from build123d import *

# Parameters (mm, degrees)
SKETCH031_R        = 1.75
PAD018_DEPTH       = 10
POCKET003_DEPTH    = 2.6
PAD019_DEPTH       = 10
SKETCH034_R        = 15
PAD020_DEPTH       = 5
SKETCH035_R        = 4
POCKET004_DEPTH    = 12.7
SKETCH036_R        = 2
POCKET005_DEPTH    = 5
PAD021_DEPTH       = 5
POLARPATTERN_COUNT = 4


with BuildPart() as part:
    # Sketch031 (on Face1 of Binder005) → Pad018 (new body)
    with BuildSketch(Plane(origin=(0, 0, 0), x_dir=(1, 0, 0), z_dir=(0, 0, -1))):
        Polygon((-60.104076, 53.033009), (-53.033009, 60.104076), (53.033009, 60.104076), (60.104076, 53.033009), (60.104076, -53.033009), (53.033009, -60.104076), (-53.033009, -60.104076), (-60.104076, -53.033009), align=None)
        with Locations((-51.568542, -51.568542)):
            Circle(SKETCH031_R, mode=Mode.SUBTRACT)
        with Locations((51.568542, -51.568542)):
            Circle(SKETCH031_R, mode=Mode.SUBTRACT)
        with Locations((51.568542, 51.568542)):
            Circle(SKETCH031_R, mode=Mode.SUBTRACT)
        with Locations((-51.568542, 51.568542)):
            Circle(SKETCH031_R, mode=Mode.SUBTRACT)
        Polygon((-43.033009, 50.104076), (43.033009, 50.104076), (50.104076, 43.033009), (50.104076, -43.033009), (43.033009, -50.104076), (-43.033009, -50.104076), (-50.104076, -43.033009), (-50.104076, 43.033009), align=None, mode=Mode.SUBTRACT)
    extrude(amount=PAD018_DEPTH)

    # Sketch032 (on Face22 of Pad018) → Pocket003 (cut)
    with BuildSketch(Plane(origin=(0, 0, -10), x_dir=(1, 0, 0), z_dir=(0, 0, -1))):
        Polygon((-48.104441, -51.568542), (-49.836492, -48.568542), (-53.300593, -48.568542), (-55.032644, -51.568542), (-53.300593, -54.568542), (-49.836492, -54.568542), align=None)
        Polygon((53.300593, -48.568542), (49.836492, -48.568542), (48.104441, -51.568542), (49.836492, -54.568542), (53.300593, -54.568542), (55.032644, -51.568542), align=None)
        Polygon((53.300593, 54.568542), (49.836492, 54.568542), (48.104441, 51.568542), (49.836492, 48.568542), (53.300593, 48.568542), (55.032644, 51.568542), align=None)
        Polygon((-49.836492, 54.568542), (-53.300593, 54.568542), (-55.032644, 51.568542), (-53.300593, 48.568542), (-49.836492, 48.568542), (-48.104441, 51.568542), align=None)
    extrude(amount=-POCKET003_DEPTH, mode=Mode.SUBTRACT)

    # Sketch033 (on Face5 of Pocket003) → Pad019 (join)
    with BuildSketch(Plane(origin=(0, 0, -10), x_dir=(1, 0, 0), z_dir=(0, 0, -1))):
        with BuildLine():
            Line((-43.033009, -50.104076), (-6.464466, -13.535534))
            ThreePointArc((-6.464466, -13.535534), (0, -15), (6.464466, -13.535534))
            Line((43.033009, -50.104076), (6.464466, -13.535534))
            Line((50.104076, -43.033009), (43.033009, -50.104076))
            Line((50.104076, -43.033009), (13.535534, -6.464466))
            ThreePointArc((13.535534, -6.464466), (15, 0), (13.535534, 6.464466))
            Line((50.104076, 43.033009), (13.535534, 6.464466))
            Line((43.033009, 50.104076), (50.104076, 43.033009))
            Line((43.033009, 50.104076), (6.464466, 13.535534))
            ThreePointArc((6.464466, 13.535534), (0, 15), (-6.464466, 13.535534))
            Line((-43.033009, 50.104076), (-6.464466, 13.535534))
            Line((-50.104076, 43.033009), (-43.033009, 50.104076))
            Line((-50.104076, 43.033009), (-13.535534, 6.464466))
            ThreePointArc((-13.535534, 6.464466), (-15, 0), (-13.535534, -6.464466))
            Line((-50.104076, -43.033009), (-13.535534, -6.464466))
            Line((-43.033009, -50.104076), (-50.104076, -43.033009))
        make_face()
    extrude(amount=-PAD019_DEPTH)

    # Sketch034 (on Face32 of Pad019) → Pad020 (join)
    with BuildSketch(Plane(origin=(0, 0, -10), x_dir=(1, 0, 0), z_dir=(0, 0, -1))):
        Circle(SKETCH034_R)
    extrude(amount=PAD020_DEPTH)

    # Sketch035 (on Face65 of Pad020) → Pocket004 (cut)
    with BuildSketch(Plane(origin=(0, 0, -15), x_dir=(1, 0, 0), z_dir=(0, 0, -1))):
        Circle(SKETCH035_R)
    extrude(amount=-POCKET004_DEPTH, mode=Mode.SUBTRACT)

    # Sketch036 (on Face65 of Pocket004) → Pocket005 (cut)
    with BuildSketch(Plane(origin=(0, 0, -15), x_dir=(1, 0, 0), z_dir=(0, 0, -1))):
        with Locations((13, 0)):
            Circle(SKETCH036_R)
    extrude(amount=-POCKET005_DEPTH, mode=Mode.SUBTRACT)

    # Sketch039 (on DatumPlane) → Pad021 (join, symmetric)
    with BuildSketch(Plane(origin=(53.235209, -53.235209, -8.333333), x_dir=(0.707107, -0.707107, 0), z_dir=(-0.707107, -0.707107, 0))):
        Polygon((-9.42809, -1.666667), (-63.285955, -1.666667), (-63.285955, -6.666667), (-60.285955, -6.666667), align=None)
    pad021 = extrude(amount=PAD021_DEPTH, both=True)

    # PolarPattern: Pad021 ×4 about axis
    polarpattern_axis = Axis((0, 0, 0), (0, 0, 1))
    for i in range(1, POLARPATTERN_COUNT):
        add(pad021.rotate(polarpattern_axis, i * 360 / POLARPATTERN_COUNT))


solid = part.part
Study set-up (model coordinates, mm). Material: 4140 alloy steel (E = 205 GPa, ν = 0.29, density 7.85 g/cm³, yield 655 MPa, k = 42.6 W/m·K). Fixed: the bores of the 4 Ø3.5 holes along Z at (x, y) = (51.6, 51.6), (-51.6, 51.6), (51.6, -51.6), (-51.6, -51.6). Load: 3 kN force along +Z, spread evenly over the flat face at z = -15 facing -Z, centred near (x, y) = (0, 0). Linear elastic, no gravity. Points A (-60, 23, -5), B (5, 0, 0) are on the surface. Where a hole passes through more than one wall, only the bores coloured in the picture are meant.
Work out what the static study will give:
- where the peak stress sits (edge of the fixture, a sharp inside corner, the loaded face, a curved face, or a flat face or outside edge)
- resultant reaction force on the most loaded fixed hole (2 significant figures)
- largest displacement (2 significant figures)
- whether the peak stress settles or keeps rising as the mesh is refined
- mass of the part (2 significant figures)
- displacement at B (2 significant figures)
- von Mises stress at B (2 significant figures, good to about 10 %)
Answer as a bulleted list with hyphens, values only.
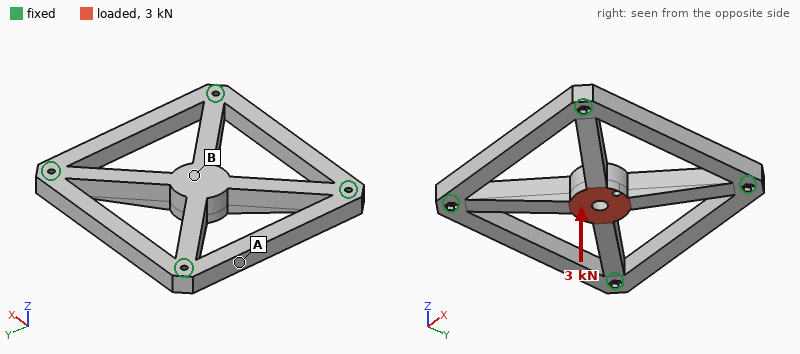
- a sharp inside corner
- 1.4 kN
- 59 µm
- keeps rising
- 620 g
- 59 µm
- 33 MPa
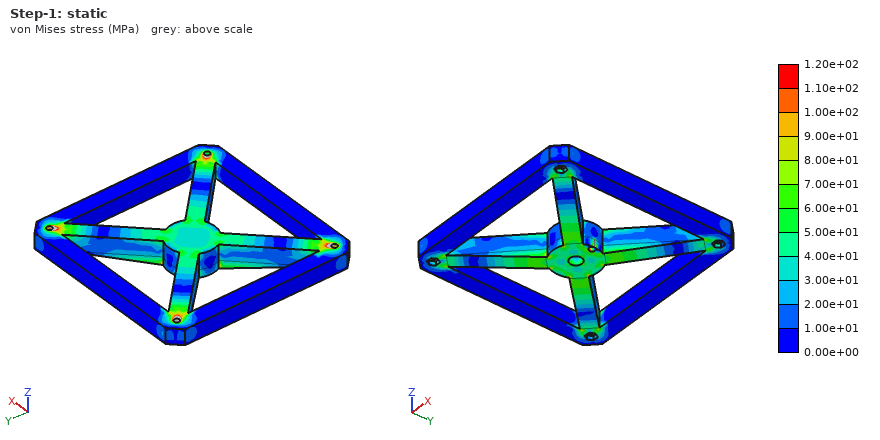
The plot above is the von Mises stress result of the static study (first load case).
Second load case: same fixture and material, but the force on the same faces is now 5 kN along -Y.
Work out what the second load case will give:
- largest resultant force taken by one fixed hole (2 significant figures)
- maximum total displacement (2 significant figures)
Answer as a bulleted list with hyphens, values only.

- 1.7 kN
- 12 µm
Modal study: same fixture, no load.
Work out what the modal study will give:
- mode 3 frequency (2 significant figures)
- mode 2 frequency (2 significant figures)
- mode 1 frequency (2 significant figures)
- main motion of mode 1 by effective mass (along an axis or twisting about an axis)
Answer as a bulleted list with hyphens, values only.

- 4300 Hz
- 4100 Hz
- 2700 Hz
- along Z
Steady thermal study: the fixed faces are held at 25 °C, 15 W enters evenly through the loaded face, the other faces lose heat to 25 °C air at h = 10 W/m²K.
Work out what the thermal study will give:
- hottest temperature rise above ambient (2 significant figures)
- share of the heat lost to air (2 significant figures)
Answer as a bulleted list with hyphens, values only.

- 41 K
- 20 %
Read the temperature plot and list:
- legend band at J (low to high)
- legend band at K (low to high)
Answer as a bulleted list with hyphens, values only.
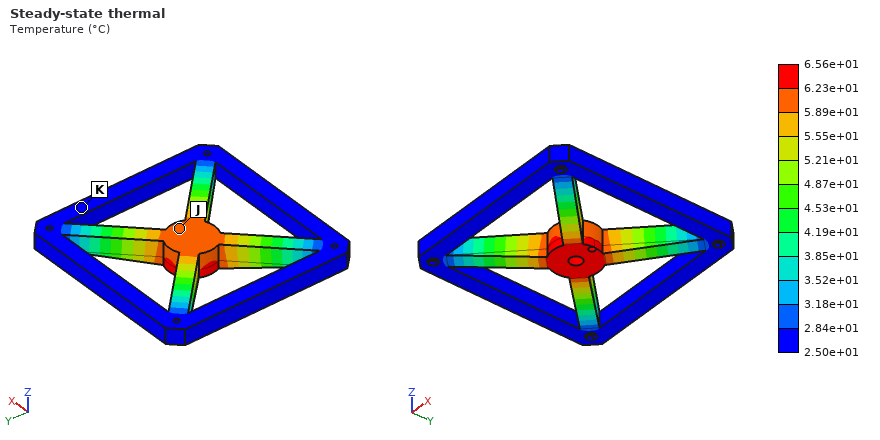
- 5.89e+01 to 6.23e+01 °C
- 2.50e+01 to 2.84e+01 °C
